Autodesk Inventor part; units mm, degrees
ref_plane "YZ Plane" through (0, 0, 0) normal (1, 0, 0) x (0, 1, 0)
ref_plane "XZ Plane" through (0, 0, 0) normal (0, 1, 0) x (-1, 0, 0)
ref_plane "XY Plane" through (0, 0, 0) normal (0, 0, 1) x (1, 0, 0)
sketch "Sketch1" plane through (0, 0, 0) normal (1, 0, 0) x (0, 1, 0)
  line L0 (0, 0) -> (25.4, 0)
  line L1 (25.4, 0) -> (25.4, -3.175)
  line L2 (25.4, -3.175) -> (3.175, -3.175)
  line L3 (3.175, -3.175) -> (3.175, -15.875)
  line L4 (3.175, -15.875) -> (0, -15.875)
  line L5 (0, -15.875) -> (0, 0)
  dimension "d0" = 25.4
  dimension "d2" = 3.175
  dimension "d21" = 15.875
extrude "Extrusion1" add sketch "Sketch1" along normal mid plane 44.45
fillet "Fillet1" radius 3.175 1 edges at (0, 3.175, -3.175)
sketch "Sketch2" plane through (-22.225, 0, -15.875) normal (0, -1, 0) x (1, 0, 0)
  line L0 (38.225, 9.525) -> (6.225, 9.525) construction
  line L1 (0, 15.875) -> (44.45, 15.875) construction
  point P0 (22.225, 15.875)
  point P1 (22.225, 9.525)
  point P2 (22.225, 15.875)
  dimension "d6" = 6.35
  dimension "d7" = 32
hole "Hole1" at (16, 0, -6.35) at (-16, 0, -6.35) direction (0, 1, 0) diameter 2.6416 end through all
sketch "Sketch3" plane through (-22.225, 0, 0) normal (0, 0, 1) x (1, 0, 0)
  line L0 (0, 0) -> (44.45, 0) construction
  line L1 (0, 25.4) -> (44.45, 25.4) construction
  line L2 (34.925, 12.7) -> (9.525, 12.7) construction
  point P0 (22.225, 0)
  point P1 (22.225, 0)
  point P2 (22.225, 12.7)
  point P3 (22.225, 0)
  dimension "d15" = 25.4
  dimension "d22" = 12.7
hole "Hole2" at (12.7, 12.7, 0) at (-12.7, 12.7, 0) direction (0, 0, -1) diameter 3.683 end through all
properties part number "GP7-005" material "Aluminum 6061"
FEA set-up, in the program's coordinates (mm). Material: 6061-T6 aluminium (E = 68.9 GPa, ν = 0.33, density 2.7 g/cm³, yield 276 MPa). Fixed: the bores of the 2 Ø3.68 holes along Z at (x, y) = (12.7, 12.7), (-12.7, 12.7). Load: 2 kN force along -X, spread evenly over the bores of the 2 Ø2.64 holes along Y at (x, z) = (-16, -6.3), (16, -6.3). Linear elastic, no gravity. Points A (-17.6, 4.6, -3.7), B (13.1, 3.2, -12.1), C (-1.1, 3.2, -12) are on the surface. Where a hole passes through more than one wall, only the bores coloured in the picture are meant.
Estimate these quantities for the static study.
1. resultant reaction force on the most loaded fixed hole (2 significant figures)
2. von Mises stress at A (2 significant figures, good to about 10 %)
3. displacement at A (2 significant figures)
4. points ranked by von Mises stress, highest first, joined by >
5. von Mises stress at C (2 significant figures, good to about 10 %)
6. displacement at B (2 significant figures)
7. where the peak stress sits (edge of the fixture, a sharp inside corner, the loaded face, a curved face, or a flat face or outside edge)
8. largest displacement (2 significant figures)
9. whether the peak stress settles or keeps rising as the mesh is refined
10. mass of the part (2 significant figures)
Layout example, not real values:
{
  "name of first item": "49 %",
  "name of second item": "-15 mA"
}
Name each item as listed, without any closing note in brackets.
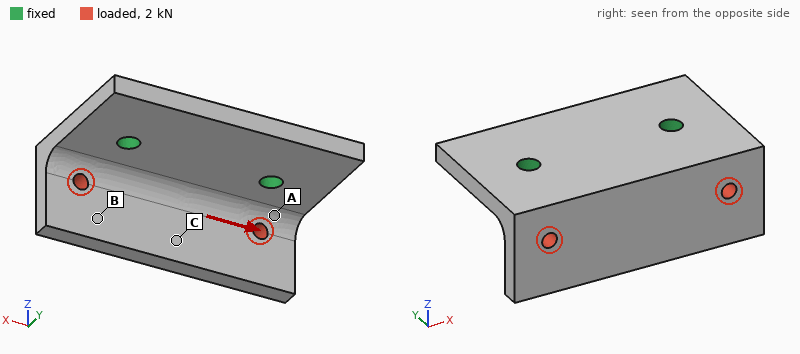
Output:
{
  "resultant reaction force on the most loaded fixed hole": "1.3 kN",
  "von Mises stress at A": "39 MPa",
  "displacement at A": "22 µm",
  "points ranked by von Mises stress, highest first, joined by >": "A > C > B",
  "von Mises stress at C": "20 MPa",
  "displacement at B": "36 µm",
  "where the peak stress sits": "edge of the fixture",
  "largest displacement": "53 µm",
  "whether the peak stress settles or keeps rising as the mesh is refined": "keeps rising",
  "mass of the part": "14 g"
}
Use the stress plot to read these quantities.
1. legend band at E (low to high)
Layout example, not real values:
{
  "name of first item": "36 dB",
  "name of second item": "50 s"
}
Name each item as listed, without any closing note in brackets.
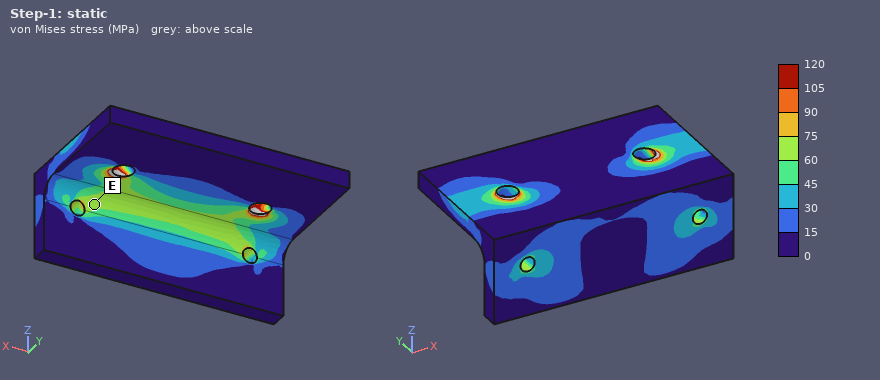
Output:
{
  "legend band at E": "60 to 75 MPa"
}
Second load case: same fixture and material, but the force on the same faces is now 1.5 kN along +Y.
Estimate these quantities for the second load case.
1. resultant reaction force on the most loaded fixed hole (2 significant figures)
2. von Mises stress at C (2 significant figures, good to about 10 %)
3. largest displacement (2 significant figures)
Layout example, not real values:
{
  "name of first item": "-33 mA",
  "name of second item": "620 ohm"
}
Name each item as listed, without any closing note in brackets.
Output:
{
  "resultant reaction force on the most loaded fixed hole": "750 N",
  "von Mises stress at C": "19 MPa",
  "largest displacement": "0.15 mm"
}
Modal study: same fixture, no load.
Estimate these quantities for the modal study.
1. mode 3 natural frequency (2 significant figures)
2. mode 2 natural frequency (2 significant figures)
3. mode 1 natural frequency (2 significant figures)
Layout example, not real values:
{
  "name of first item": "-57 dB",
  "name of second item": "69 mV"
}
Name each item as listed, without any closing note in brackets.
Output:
{
  "mode 3 natural frequency": "14 kHz",
  "mode 2 natural frequency": "8300 Hz",
  "mode 1 natural frequency": "5500 Hz"
}
